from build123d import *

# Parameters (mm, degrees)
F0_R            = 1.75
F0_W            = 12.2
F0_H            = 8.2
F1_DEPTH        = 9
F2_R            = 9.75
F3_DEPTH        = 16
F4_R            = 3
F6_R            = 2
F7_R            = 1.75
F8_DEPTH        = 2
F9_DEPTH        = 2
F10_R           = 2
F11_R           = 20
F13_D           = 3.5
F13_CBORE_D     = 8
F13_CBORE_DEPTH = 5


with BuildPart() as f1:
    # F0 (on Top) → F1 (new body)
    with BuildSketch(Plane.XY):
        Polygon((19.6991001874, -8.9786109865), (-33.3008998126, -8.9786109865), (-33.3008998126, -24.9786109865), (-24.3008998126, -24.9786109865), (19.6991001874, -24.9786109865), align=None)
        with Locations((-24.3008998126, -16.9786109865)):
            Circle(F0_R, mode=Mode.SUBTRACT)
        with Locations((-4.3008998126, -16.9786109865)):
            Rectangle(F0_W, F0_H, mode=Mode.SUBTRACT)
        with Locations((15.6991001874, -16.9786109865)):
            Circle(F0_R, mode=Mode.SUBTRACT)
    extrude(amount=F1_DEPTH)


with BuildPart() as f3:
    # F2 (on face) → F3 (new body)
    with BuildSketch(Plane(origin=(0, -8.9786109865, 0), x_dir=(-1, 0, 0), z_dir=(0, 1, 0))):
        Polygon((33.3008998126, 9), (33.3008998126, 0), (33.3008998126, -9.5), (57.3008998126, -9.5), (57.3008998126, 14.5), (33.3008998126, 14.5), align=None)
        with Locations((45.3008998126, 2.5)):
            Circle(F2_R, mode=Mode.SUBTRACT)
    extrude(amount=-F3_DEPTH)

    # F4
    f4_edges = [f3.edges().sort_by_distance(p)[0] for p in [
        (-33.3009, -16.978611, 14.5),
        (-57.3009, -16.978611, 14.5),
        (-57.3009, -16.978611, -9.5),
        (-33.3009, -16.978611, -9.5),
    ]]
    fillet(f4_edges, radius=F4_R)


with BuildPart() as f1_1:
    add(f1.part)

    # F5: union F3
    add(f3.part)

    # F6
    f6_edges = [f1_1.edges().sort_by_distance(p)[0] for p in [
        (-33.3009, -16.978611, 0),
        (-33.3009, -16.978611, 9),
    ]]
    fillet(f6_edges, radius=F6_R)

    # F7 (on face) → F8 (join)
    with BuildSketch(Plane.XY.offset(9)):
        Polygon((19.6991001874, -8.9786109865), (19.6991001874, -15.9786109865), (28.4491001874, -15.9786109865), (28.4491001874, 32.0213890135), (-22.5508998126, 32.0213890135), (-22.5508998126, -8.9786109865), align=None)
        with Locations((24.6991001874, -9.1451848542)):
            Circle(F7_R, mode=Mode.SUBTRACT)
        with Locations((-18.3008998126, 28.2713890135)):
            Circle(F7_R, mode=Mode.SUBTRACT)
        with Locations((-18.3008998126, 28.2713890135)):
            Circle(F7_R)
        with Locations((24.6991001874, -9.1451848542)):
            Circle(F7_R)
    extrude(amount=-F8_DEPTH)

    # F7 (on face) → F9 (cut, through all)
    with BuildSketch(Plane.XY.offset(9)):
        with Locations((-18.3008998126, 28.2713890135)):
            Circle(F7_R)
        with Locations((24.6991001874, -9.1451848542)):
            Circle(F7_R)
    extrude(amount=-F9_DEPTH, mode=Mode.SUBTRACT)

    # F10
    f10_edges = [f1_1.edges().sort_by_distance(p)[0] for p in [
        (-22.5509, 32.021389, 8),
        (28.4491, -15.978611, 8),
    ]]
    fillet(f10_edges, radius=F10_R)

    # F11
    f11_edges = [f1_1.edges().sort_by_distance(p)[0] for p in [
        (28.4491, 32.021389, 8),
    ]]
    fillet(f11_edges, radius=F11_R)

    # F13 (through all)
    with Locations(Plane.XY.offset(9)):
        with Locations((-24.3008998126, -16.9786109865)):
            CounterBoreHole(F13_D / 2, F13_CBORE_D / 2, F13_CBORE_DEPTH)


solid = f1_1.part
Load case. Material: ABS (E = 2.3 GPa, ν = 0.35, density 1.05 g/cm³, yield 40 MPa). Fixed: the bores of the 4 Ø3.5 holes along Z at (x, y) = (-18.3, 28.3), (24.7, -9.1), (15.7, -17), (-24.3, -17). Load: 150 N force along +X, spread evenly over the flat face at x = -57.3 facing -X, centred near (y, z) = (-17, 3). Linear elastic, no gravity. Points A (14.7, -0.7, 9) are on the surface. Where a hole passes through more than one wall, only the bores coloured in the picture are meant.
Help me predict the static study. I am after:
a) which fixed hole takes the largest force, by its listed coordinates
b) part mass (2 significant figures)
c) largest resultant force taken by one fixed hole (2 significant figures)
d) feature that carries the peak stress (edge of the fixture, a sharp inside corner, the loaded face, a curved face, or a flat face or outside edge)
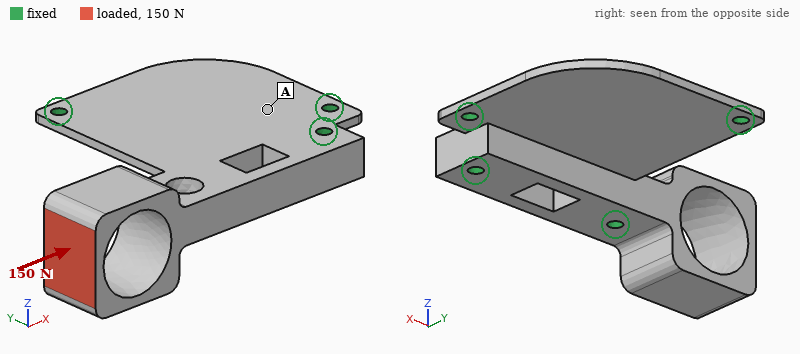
(-24.3, -17)
16 g
130 N
a curved face
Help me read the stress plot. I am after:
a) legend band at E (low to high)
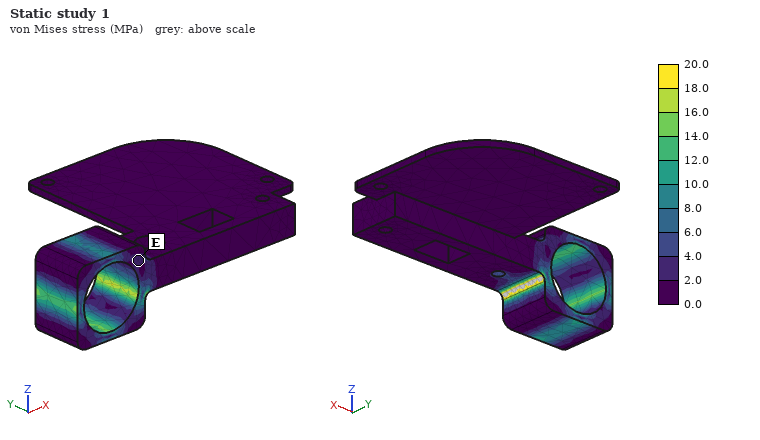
2.0 to 4.0 MPa
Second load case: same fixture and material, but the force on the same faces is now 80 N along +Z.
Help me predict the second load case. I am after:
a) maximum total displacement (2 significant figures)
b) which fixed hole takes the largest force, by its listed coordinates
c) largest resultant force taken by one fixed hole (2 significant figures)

1.2 mm
(-24.3, -17)
170 N
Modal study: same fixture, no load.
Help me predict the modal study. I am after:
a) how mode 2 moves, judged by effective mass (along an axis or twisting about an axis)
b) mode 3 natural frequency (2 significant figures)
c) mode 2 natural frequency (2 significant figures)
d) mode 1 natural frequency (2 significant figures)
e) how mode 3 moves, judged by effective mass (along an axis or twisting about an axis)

along Z
1400 Hz
890 Hz
620 Hz
along Y
